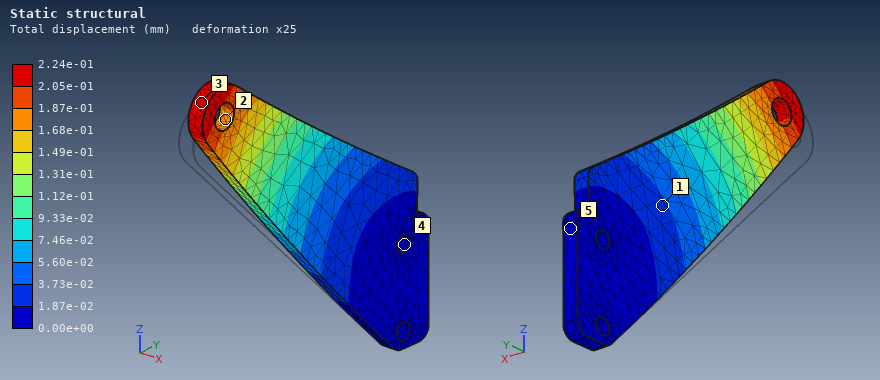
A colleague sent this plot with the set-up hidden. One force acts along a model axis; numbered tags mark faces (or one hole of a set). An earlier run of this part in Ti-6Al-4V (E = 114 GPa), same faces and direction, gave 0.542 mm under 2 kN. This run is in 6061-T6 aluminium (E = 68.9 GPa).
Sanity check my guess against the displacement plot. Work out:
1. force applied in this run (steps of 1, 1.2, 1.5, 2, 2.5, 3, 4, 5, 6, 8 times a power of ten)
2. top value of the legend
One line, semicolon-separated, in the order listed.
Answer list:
500 N; 2.24e-01 mm
